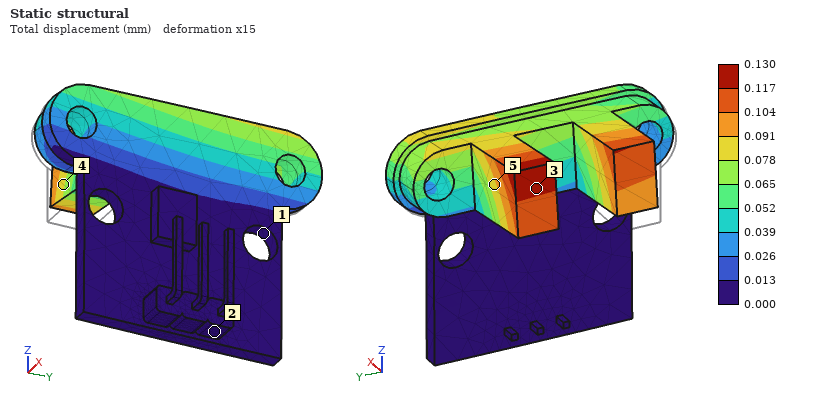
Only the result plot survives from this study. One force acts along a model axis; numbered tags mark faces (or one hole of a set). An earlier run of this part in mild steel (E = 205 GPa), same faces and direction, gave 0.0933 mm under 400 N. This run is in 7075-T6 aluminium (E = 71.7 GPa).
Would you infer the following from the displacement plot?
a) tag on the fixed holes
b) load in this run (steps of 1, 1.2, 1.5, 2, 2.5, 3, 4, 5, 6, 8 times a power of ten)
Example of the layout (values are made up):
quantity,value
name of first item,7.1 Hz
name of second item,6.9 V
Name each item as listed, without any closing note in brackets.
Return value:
quantity,value
tag on the fixed holes,1
load in this run,200 N
